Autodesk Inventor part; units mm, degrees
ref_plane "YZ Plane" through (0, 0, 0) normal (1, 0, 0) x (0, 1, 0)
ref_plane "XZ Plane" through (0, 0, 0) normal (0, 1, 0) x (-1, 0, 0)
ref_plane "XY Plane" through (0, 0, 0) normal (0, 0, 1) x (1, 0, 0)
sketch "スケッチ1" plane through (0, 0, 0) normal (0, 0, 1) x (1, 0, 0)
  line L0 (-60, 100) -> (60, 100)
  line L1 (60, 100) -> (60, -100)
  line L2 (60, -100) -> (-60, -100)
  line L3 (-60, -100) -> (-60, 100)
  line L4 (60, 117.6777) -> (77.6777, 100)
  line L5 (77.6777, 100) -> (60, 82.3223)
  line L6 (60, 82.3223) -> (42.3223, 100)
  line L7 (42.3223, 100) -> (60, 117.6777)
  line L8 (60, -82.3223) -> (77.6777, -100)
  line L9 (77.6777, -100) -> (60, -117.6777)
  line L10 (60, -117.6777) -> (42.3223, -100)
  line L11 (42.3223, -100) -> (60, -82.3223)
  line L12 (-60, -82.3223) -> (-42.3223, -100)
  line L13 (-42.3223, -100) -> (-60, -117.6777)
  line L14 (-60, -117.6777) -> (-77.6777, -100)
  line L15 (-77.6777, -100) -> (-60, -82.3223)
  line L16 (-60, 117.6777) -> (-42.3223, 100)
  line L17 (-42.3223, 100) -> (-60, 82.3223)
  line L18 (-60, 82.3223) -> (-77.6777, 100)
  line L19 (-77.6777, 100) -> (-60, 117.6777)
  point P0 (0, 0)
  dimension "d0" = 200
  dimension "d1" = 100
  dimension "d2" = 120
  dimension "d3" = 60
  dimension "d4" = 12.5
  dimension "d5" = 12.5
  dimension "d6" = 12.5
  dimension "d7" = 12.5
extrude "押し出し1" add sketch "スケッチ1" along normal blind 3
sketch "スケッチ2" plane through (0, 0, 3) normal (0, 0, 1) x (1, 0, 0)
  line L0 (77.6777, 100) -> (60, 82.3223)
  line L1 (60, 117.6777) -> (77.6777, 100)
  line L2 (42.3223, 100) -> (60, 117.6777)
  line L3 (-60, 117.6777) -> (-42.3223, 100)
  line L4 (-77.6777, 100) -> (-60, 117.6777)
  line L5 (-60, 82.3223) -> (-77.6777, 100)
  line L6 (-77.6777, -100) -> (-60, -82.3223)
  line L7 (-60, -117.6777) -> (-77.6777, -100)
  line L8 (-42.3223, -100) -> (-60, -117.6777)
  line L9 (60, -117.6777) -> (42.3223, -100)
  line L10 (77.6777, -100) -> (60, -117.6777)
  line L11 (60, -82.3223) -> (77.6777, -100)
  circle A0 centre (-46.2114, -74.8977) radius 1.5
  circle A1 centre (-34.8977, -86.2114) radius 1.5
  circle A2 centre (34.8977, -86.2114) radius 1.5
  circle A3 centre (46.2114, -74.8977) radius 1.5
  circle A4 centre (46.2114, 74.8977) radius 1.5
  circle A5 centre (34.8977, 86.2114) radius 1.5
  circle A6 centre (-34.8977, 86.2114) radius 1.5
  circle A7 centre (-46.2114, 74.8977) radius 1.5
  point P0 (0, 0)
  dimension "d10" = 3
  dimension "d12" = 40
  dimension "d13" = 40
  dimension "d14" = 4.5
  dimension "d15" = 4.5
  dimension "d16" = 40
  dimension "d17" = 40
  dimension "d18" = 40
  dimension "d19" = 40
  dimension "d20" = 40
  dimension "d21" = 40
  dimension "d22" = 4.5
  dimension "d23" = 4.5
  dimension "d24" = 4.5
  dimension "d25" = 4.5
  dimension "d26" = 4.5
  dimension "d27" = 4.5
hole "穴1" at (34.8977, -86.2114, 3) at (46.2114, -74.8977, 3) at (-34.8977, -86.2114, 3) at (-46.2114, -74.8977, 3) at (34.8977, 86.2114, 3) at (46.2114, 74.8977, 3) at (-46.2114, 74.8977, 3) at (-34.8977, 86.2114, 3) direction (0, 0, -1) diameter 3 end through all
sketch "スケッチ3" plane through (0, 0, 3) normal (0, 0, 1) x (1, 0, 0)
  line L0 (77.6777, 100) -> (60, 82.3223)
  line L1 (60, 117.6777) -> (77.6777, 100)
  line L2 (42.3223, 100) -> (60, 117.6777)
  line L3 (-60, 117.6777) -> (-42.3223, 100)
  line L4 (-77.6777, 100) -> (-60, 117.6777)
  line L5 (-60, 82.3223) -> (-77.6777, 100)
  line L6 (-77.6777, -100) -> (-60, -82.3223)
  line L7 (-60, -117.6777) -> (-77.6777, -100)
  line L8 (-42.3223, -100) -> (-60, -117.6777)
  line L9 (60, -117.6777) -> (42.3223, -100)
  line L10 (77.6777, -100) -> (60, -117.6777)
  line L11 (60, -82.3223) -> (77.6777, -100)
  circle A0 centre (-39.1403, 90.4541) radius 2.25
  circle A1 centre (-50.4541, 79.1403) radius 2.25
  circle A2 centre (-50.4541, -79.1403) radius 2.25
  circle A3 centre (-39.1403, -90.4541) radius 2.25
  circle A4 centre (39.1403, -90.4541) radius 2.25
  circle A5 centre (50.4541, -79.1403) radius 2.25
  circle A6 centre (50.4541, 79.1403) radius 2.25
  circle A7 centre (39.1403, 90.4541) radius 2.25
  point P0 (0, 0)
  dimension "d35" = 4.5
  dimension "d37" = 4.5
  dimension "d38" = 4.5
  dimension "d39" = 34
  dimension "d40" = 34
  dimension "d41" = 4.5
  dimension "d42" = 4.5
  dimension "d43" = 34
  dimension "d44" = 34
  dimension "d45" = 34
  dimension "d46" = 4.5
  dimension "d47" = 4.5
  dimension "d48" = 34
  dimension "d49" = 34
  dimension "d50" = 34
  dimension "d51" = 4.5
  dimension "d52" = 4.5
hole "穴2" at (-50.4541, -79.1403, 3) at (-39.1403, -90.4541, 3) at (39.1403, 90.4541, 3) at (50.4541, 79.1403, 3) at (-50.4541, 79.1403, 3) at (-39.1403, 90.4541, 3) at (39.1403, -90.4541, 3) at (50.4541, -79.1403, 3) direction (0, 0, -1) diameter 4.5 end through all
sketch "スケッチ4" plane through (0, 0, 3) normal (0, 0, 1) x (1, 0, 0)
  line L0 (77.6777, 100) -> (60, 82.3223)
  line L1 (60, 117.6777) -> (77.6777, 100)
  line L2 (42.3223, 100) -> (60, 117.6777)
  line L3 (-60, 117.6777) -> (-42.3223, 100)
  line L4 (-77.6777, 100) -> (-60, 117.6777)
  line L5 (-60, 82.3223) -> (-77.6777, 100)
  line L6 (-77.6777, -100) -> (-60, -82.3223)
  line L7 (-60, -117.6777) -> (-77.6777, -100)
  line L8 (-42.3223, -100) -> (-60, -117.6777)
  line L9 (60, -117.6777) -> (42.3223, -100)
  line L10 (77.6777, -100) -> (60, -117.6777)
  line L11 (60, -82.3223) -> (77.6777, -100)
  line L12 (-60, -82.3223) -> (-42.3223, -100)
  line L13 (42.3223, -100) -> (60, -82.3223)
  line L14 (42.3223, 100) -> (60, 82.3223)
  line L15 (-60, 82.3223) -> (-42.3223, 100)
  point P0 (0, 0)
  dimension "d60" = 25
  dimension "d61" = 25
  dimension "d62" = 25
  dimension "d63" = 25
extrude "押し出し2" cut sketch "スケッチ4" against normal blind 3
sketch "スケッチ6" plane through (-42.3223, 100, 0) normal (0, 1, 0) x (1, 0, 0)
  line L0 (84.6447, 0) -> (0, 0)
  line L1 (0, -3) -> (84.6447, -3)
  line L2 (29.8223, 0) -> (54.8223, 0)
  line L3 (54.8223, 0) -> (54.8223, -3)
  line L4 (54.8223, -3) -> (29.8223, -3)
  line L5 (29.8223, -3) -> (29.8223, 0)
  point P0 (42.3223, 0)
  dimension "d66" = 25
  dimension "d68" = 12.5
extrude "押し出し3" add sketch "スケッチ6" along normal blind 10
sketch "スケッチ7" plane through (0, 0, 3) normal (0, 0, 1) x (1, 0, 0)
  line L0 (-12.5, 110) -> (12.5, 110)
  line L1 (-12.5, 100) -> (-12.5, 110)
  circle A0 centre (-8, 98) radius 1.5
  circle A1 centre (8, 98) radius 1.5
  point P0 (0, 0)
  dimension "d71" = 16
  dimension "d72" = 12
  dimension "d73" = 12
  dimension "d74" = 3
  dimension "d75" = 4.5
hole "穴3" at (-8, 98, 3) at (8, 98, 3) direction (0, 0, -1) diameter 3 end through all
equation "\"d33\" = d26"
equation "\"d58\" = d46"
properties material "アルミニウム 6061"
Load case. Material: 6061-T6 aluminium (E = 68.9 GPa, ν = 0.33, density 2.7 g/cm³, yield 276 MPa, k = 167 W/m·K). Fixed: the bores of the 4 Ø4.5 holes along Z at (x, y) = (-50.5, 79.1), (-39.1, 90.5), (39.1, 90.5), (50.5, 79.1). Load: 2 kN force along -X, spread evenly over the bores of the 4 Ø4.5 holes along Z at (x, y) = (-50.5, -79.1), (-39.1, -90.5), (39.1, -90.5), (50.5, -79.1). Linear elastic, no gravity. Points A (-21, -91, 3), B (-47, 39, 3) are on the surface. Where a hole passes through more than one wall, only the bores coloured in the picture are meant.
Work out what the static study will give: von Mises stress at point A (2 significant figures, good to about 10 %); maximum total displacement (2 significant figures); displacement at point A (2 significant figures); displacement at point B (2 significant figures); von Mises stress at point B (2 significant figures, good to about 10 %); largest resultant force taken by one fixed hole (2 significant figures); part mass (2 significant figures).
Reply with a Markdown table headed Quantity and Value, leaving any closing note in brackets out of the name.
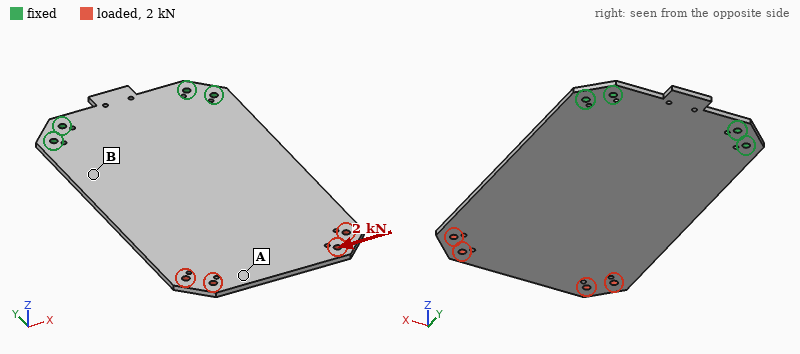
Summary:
| Quantity | Value |
|---|---|
| von Mises stress at point A | 7.2 MPa |
| maximum total displacement | 0.18 mm |
| displacement at point A | 0.16 mm |
| displacement at point B | 0.033 mm |
| von Mises stress at point B | 28 MPa |
| largest resultant force taken by one fixed hole | 2.6 kN |
| part mass | 190 g |
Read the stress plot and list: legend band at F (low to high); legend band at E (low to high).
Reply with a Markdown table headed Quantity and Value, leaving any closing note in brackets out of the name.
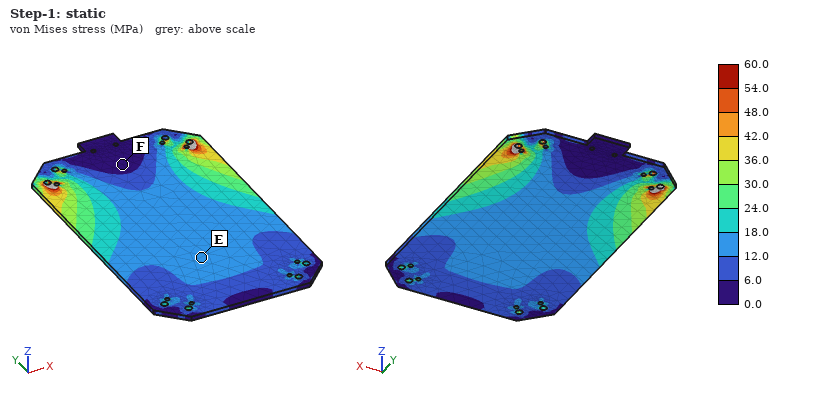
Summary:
| Quantity | Value |
|---|---|
| legend band at F | 0.0 to 6.0 MPa |
| legend band at E | 12.0 to 18.0 MPa |
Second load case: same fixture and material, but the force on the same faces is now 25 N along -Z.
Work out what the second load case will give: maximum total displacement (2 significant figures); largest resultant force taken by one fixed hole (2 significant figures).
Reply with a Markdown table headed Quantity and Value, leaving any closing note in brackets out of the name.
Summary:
| Quantity | Value |
|---|---|
| maximum total displacement | 2.5 mm |
| largest resultant force taken by one fixed hole | 54 N |
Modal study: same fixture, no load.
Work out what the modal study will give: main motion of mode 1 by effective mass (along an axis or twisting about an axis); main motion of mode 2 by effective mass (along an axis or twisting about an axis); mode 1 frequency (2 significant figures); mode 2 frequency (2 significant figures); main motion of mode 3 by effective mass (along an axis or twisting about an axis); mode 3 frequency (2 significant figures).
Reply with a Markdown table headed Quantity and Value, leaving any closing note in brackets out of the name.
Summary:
| Quantity | Value |
|---|---|
| main motion of mode 1 by effective mass | along Z |
| main motion of mode 2 by effective mass | twisting about Y |
| mode 1 frequency | 73 Hz |
| mode 2 frequency | 270 Hz |
| main motion of mode 3 by effective mass | along Z |
| mode 3 frequency | 460 Hz |
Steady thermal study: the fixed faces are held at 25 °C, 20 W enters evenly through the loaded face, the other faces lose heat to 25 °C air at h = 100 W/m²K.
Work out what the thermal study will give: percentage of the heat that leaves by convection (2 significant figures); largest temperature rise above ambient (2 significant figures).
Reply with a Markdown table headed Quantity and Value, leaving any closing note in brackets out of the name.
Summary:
| Quantity | Value |
|---|---|
| percentage of the heat that leaves by convection | 96 % |
| largest temperature rise above ambient | 18 K |
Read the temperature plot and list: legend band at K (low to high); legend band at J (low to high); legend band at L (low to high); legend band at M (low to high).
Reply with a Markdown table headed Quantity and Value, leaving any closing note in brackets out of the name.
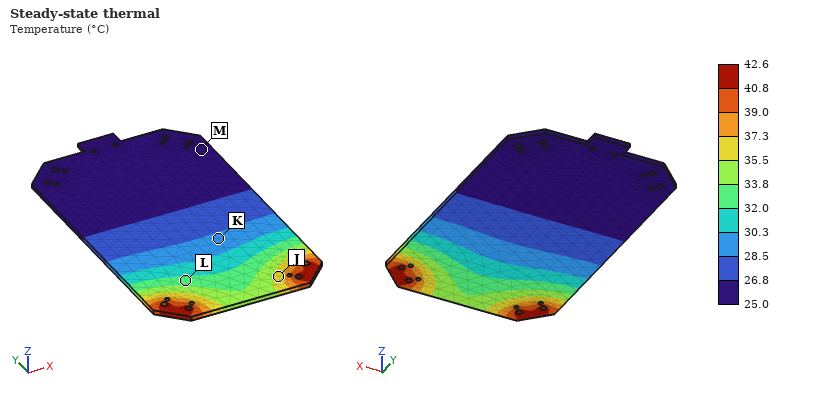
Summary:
| Quantity | Value |
|---|---|
| legend band at K | 28.5 to 30.3 °C |
| legend band at J | 35.5 to 37.3 °C |
| legend band at L | 32.0 to 33.8 °C |
| legend band at M | 25.0 to 26.8 °C |
